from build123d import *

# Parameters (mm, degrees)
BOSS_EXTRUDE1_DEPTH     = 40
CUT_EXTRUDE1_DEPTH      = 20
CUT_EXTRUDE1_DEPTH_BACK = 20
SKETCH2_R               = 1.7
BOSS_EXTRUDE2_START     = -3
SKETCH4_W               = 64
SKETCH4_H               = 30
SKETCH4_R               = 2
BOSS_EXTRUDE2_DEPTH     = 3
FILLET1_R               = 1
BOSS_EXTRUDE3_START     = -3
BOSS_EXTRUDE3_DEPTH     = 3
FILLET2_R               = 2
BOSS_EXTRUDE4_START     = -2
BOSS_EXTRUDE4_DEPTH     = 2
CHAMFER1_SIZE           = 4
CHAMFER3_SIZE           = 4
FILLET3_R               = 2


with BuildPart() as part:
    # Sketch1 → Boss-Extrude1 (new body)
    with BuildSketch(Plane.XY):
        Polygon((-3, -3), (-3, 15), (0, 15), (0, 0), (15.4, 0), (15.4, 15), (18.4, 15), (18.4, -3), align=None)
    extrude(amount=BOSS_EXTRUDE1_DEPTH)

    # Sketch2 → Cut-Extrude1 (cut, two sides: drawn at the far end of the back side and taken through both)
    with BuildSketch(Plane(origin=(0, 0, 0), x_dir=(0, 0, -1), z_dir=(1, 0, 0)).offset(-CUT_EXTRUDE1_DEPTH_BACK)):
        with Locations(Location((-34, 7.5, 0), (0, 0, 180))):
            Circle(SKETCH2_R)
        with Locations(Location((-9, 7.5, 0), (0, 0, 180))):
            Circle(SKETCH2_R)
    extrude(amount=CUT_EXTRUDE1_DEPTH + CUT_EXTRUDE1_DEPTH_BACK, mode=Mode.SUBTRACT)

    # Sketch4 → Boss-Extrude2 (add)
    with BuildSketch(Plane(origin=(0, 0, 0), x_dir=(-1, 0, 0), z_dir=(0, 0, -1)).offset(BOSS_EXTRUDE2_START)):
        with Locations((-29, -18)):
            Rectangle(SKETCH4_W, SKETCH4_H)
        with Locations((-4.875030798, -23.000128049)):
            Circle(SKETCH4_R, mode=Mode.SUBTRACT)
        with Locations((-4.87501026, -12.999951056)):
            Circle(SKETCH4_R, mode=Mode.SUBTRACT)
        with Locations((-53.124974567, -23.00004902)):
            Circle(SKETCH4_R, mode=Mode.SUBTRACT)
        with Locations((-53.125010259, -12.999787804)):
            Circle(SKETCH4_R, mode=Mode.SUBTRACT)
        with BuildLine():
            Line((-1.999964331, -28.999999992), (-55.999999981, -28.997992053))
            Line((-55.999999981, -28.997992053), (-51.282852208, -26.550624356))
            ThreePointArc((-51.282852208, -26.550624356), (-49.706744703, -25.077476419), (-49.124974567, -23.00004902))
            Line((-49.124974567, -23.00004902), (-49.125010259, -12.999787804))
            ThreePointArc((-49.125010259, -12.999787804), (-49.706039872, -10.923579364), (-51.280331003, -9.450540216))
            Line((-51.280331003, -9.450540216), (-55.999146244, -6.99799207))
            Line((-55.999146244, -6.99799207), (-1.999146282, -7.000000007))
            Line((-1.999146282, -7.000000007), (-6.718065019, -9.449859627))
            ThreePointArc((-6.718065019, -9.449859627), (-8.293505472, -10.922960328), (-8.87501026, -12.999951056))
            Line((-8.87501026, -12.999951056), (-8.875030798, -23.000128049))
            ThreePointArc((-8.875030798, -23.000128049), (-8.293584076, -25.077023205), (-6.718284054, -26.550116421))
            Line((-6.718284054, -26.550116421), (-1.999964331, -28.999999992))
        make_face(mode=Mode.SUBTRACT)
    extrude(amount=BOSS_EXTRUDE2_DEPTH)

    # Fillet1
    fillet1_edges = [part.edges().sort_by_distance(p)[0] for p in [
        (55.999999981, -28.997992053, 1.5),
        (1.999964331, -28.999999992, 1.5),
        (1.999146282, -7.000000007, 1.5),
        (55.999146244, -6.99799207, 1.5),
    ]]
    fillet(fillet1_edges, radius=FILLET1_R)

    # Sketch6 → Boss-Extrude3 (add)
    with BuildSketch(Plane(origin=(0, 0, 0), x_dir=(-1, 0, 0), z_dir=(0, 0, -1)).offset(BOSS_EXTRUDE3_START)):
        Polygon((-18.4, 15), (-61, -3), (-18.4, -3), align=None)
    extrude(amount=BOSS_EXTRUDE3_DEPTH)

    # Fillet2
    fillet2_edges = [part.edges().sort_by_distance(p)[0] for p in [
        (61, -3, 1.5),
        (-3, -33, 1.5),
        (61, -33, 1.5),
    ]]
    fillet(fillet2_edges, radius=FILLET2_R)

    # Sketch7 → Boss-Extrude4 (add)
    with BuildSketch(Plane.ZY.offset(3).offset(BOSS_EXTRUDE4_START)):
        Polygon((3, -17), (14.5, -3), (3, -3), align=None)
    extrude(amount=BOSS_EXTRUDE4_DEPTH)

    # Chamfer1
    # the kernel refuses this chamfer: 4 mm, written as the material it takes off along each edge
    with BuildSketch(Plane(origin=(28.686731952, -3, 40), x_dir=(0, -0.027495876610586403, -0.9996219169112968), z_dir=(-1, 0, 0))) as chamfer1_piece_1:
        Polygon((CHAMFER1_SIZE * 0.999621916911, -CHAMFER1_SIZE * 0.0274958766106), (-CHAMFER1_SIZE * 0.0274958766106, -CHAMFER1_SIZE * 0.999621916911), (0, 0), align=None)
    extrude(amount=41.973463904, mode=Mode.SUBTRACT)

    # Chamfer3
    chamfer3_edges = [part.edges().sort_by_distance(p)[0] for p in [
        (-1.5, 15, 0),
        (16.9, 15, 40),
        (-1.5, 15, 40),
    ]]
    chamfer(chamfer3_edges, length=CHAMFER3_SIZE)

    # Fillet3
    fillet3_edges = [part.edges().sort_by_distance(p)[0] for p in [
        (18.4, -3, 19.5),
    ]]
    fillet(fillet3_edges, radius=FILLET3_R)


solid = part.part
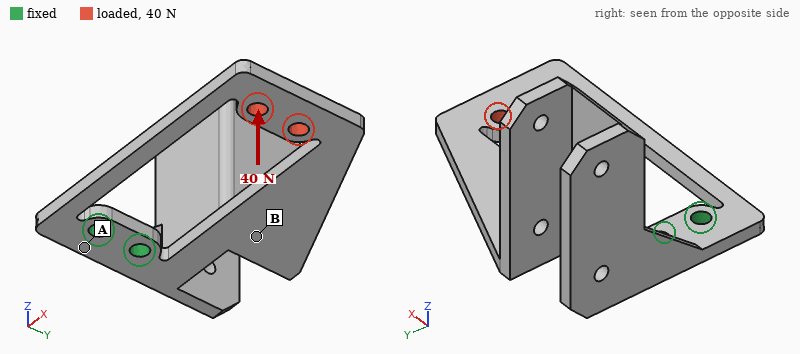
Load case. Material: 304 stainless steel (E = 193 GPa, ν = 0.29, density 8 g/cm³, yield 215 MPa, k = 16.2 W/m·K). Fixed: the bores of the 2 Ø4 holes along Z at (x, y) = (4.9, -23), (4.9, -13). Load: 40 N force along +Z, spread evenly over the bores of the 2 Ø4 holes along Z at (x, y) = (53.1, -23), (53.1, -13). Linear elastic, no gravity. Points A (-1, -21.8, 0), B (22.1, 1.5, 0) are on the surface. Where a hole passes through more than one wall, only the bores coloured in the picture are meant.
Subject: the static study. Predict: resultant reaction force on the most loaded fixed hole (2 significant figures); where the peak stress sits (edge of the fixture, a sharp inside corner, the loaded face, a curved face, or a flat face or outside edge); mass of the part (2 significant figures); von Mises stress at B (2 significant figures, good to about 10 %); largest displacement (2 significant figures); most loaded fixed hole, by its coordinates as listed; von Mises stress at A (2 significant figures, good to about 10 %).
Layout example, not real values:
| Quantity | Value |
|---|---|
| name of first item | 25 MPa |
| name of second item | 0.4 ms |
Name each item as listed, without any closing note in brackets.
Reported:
| Quantity | Value |
|---|---|
| resultant reaction force on the most loaded fixed hole | 33 N |
| where the peak stress sits | a curved face |
| mass of the part | 79 g |
| von Mises stress at B | 32 MPa |
| largest displacement | 0.30 mm |
| most loaded fixed hole, by its coordinates as listed | (4.9, -23) |
| von Mises stress at A | 12 MPa |
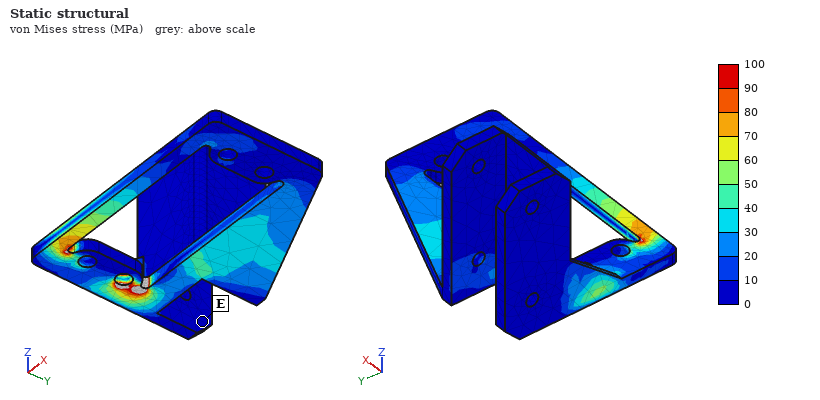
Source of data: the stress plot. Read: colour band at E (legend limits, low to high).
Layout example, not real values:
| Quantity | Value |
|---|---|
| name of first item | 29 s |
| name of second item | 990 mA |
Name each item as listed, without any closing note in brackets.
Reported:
| Quantity | Value |
|---|---|
| colour band at E | 0 to 10 MPa |
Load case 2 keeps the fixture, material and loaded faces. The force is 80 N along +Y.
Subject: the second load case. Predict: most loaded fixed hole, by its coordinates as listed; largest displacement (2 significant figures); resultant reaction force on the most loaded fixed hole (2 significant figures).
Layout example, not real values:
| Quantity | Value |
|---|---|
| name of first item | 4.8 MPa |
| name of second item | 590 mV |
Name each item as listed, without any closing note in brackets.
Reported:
| Quantity | Value |
|---|---|
| most loaded fixed hole, by its coordinates as listed | (4.9, -13) |
| largest displacement | 72 µm |
| resultant reaction force on the most loaded fixed hole | 290 N |
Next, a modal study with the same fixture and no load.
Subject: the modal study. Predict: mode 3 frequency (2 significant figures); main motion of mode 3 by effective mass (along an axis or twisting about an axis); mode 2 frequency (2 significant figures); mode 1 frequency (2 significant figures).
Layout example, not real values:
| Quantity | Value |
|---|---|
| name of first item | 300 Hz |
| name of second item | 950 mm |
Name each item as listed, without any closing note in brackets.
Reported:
| Quantity | Value |
|---|---|
| mode 3 frequency | 1200 Hz |
| main motion of mode 3 by effective mass | along X |
| mode 2 frequency | 950 Hz |
| mode 1 frequency | 540 Hz |
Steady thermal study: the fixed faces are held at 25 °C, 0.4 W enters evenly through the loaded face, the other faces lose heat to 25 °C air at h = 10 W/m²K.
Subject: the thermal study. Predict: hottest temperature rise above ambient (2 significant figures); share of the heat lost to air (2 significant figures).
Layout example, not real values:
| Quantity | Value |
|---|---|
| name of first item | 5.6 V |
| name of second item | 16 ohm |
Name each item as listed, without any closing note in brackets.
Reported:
| Quantity | Value |
|---|---|
| hottest temperature rise above ambient | 19 K |
| share of the heat lost to air | 76 % |
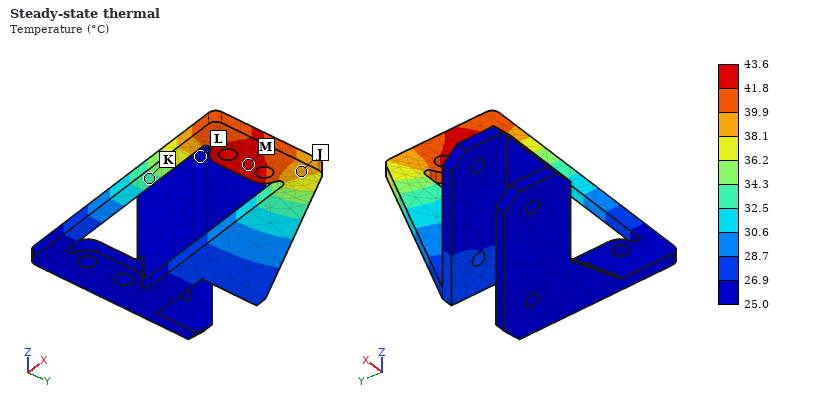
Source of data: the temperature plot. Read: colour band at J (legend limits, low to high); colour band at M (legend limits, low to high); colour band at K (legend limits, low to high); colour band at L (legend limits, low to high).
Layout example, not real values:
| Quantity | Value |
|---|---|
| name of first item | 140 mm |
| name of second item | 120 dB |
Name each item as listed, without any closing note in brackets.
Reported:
| Quantity | Value |
|---|---|
| colour band at J | 38.1 to 39.9 °C |
| colour band at M | 41.8 to 43.6 °C |
| colour band at K | 32.5 to 34.3 °C |
| colour band at L | 25.0 to 26.9 °C |
